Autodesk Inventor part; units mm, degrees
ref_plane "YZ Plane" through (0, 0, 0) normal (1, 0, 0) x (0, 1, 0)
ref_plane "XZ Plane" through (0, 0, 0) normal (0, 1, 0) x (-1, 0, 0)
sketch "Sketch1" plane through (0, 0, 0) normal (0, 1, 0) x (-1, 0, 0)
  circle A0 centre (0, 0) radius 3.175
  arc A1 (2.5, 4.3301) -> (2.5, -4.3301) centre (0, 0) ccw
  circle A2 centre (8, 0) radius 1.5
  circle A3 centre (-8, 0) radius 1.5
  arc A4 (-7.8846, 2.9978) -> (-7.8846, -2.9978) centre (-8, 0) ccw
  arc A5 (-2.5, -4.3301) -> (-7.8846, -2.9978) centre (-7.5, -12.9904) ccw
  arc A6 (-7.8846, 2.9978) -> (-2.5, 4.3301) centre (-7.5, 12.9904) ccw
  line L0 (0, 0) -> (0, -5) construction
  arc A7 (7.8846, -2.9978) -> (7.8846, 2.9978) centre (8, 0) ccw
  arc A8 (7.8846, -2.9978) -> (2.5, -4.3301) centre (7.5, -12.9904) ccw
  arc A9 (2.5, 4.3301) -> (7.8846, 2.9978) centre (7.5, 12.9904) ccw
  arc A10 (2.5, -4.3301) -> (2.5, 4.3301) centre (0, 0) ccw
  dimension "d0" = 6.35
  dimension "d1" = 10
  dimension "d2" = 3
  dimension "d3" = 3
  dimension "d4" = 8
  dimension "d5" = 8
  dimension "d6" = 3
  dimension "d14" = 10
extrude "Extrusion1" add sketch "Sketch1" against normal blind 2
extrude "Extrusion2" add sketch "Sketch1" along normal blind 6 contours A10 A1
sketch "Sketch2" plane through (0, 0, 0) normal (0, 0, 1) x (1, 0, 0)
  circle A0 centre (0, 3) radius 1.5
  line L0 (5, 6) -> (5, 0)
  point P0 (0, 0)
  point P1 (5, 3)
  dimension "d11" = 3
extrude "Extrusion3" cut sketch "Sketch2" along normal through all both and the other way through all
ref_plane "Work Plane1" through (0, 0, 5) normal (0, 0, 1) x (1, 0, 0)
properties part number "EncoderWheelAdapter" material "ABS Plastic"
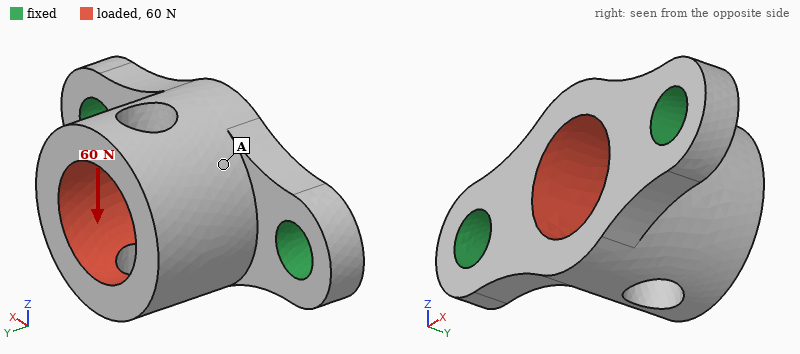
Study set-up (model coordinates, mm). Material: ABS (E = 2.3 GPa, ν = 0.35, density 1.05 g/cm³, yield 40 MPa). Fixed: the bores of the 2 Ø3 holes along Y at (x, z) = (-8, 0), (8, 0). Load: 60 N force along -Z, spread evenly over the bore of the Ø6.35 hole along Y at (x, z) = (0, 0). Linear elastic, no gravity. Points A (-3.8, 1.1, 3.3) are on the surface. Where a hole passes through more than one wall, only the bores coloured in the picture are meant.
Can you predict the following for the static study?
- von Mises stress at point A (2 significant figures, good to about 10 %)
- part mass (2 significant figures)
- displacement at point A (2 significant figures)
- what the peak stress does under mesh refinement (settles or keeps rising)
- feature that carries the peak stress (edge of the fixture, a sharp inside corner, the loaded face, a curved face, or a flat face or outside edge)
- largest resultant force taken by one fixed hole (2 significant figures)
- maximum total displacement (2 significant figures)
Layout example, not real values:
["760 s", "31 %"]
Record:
["3.6 MPa", "0.49 g", "0.071 mm", "keeps rising", "edge of the fixture", "30 N", "0.16 mm"]
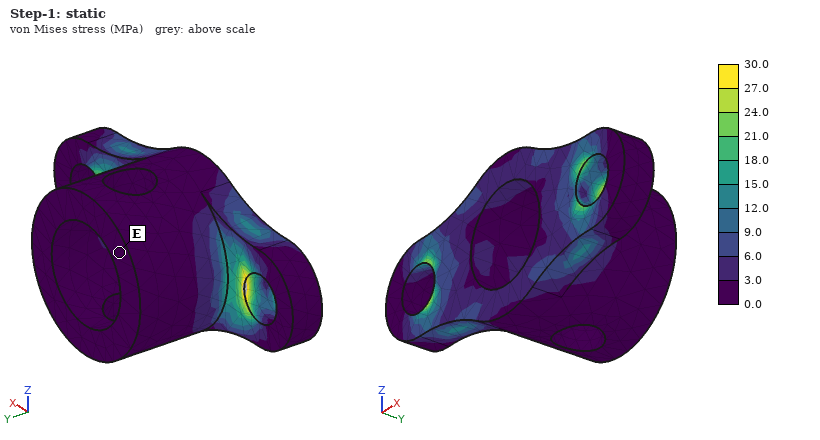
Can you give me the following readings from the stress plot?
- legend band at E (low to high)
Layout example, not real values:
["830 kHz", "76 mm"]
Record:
["0.0 to 3.0 MPa"]
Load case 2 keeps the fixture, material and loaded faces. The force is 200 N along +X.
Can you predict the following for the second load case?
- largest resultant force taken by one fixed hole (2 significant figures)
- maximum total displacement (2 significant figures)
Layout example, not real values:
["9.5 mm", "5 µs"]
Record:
["110 N", "89 µm"]
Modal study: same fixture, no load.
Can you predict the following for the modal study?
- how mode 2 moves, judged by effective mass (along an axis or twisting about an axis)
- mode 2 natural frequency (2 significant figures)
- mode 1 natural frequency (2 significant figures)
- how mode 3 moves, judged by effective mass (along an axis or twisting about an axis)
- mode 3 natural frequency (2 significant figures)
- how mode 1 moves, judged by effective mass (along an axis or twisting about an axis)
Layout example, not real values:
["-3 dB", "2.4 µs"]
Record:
["along Y", "12 kHz", "5500 Hz", "along X", "14 kHz", "along Z"]
